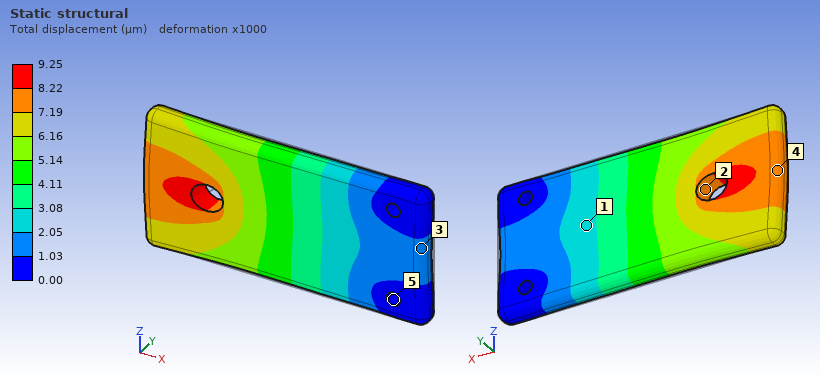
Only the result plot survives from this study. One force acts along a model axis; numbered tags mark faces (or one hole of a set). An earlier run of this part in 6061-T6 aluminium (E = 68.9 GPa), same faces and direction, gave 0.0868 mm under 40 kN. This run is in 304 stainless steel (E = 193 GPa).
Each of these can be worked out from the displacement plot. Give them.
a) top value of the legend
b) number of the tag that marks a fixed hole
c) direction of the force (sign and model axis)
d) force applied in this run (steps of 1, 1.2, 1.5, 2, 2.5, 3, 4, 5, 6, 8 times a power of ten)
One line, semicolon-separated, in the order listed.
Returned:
9.25 µm; 5; -X; 12 kN
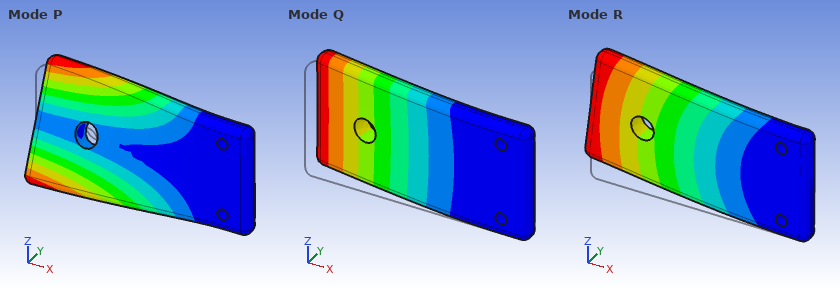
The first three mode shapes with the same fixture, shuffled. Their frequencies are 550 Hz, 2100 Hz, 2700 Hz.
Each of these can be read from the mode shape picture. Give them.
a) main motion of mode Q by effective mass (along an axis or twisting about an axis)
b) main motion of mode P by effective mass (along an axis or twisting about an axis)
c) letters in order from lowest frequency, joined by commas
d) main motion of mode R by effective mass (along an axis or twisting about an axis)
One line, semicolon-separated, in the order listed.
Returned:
along Y; twisting about X; Q, P, R; along Z
